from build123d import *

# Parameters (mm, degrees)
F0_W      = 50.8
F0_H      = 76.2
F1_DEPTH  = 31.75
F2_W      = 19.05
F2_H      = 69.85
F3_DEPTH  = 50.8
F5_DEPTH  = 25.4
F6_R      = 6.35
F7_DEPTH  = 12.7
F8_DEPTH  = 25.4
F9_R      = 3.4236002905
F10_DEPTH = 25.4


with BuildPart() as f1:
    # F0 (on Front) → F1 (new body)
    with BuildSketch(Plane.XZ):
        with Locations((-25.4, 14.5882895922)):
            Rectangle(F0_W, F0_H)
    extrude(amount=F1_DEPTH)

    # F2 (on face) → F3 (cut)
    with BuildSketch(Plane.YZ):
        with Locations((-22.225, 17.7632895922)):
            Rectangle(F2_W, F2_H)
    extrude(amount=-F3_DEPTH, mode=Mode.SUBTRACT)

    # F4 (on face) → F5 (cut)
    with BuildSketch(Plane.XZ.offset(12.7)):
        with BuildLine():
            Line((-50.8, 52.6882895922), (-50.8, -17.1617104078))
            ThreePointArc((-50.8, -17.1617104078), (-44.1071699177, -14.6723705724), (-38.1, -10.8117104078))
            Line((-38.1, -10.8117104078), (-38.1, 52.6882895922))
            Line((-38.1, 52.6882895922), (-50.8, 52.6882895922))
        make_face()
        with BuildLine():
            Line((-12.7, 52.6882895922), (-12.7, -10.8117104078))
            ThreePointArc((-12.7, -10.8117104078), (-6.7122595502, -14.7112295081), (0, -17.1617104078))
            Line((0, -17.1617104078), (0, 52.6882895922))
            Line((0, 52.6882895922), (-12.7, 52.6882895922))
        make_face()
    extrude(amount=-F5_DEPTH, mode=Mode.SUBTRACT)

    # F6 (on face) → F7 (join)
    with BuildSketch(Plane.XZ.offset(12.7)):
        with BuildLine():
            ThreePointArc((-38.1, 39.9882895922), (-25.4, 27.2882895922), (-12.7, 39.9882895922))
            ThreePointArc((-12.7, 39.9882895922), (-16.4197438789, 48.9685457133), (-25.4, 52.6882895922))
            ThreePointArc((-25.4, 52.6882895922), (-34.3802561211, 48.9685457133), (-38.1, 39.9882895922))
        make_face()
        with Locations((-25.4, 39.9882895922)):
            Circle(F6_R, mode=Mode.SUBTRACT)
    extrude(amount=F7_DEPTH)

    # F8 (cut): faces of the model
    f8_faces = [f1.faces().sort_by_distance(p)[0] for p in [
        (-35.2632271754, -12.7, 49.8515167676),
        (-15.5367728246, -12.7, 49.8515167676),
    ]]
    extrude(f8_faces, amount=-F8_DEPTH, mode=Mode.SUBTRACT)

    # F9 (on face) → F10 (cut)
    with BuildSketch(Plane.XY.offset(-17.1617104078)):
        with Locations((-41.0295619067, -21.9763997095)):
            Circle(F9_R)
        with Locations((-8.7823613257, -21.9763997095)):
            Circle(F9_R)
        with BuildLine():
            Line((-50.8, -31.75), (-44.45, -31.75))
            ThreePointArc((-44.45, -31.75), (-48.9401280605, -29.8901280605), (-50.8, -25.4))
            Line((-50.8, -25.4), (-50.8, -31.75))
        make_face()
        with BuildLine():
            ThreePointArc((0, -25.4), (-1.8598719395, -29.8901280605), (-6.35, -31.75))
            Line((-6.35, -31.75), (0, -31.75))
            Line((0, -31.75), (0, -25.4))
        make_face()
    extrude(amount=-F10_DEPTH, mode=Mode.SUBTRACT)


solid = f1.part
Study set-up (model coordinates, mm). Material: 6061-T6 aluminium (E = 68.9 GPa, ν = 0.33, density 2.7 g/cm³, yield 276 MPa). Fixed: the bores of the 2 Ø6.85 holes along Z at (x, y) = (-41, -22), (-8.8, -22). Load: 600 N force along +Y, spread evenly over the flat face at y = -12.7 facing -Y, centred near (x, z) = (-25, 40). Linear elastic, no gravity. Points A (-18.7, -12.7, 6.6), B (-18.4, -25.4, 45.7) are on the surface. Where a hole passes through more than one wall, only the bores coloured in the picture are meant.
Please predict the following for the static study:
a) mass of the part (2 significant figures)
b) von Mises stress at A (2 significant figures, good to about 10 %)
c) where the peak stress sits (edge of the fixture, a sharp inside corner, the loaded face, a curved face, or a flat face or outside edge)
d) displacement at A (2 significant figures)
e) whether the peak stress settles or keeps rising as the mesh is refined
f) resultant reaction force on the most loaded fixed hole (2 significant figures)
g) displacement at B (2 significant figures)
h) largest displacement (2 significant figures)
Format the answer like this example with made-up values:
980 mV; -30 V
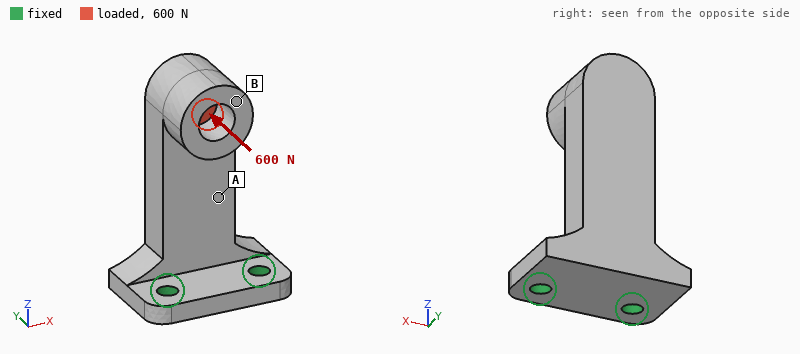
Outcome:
100 g; 29 MPa; edge of the fixture; 0.18 mm; keeps rising; 360 N; 0.53 mm; 0.59 mm
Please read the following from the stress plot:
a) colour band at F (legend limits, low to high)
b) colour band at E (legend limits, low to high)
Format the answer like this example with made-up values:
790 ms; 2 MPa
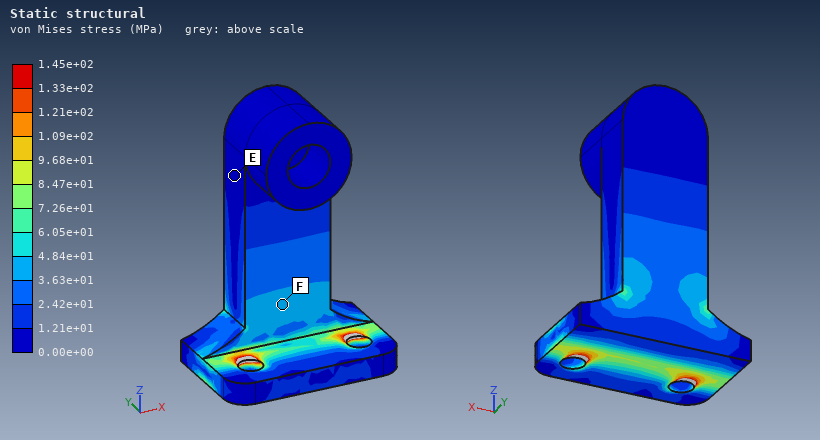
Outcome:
3.63e+01 to 4.84e+01 MPa; 0.00e+00 to 1.21e+01 MPa
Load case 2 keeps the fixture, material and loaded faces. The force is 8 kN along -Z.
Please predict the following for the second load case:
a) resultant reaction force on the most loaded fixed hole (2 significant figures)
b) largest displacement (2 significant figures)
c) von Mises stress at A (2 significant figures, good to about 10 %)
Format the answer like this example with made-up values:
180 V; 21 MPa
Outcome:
4.1 kN; 0.22 mm; 99 MPa
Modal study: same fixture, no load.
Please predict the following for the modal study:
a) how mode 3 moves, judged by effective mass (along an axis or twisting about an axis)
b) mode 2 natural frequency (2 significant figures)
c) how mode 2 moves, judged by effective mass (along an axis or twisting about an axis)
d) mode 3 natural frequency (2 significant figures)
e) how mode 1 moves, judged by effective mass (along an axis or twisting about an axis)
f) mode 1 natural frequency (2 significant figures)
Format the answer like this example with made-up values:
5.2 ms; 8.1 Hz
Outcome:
along Z; 2100 Hz; along X; 5100 Hz; along Y; 890 Hz
